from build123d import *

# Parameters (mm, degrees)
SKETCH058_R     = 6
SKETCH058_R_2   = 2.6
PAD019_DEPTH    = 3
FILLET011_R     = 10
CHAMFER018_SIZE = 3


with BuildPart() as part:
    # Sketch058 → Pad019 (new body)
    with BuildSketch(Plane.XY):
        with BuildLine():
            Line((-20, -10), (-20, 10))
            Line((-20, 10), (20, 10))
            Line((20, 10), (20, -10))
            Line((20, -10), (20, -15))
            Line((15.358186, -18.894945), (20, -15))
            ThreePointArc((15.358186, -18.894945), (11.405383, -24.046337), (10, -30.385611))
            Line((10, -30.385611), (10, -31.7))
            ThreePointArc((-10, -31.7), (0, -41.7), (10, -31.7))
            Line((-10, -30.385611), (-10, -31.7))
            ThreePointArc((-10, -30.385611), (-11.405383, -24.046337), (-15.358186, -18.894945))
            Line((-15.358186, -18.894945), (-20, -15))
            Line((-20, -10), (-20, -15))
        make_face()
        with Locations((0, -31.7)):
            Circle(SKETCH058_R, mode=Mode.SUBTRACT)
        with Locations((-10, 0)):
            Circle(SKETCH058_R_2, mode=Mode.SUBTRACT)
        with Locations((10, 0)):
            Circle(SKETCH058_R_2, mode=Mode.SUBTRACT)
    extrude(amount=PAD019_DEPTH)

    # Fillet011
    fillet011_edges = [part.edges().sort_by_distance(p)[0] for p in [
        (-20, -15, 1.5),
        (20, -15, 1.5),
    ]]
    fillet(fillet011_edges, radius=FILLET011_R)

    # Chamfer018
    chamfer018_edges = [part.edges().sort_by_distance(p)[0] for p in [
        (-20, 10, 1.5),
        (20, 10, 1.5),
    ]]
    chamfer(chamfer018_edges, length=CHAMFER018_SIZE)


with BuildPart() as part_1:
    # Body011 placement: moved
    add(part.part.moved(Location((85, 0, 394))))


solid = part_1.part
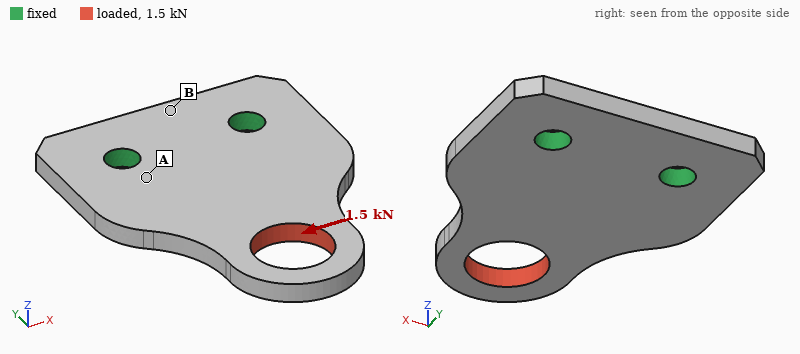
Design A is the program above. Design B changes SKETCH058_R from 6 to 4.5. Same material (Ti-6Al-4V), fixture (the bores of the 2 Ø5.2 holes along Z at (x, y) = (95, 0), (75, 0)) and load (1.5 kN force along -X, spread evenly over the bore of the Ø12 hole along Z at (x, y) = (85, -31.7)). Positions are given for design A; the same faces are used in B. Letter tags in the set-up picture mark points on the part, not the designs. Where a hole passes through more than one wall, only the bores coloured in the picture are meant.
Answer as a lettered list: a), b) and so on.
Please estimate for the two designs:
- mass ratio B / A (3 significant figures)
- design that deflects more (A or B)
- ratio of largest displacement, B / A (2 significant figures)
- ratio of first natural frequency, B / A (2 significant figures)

a) 1.03
b) A
c) 0.72
d) 0.93
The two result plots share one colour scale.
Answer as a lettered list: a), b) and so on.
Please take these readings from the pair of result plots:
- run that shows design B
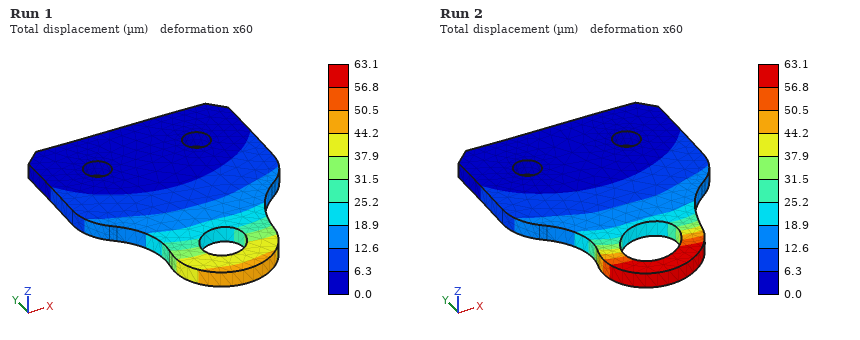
a) Run 1
